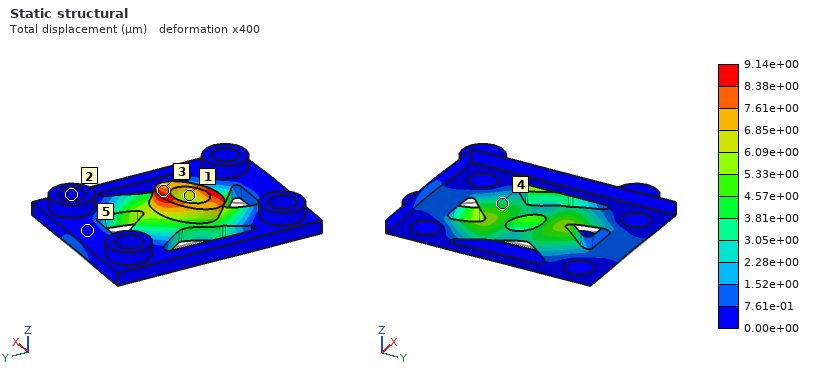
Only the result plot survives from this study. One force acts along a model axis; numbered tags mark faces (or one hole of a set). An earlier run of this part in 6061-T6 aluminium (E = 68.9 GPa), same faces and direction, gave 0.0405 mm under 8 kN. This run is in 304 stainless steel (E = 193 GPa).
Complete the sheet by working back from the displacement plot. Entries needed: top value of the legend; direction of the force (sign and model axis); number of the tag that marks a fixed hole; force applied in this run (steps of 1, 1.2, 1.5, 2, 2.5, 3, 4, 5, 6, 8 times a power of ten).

9.14e+00 µm
-Y
2
5 kN
